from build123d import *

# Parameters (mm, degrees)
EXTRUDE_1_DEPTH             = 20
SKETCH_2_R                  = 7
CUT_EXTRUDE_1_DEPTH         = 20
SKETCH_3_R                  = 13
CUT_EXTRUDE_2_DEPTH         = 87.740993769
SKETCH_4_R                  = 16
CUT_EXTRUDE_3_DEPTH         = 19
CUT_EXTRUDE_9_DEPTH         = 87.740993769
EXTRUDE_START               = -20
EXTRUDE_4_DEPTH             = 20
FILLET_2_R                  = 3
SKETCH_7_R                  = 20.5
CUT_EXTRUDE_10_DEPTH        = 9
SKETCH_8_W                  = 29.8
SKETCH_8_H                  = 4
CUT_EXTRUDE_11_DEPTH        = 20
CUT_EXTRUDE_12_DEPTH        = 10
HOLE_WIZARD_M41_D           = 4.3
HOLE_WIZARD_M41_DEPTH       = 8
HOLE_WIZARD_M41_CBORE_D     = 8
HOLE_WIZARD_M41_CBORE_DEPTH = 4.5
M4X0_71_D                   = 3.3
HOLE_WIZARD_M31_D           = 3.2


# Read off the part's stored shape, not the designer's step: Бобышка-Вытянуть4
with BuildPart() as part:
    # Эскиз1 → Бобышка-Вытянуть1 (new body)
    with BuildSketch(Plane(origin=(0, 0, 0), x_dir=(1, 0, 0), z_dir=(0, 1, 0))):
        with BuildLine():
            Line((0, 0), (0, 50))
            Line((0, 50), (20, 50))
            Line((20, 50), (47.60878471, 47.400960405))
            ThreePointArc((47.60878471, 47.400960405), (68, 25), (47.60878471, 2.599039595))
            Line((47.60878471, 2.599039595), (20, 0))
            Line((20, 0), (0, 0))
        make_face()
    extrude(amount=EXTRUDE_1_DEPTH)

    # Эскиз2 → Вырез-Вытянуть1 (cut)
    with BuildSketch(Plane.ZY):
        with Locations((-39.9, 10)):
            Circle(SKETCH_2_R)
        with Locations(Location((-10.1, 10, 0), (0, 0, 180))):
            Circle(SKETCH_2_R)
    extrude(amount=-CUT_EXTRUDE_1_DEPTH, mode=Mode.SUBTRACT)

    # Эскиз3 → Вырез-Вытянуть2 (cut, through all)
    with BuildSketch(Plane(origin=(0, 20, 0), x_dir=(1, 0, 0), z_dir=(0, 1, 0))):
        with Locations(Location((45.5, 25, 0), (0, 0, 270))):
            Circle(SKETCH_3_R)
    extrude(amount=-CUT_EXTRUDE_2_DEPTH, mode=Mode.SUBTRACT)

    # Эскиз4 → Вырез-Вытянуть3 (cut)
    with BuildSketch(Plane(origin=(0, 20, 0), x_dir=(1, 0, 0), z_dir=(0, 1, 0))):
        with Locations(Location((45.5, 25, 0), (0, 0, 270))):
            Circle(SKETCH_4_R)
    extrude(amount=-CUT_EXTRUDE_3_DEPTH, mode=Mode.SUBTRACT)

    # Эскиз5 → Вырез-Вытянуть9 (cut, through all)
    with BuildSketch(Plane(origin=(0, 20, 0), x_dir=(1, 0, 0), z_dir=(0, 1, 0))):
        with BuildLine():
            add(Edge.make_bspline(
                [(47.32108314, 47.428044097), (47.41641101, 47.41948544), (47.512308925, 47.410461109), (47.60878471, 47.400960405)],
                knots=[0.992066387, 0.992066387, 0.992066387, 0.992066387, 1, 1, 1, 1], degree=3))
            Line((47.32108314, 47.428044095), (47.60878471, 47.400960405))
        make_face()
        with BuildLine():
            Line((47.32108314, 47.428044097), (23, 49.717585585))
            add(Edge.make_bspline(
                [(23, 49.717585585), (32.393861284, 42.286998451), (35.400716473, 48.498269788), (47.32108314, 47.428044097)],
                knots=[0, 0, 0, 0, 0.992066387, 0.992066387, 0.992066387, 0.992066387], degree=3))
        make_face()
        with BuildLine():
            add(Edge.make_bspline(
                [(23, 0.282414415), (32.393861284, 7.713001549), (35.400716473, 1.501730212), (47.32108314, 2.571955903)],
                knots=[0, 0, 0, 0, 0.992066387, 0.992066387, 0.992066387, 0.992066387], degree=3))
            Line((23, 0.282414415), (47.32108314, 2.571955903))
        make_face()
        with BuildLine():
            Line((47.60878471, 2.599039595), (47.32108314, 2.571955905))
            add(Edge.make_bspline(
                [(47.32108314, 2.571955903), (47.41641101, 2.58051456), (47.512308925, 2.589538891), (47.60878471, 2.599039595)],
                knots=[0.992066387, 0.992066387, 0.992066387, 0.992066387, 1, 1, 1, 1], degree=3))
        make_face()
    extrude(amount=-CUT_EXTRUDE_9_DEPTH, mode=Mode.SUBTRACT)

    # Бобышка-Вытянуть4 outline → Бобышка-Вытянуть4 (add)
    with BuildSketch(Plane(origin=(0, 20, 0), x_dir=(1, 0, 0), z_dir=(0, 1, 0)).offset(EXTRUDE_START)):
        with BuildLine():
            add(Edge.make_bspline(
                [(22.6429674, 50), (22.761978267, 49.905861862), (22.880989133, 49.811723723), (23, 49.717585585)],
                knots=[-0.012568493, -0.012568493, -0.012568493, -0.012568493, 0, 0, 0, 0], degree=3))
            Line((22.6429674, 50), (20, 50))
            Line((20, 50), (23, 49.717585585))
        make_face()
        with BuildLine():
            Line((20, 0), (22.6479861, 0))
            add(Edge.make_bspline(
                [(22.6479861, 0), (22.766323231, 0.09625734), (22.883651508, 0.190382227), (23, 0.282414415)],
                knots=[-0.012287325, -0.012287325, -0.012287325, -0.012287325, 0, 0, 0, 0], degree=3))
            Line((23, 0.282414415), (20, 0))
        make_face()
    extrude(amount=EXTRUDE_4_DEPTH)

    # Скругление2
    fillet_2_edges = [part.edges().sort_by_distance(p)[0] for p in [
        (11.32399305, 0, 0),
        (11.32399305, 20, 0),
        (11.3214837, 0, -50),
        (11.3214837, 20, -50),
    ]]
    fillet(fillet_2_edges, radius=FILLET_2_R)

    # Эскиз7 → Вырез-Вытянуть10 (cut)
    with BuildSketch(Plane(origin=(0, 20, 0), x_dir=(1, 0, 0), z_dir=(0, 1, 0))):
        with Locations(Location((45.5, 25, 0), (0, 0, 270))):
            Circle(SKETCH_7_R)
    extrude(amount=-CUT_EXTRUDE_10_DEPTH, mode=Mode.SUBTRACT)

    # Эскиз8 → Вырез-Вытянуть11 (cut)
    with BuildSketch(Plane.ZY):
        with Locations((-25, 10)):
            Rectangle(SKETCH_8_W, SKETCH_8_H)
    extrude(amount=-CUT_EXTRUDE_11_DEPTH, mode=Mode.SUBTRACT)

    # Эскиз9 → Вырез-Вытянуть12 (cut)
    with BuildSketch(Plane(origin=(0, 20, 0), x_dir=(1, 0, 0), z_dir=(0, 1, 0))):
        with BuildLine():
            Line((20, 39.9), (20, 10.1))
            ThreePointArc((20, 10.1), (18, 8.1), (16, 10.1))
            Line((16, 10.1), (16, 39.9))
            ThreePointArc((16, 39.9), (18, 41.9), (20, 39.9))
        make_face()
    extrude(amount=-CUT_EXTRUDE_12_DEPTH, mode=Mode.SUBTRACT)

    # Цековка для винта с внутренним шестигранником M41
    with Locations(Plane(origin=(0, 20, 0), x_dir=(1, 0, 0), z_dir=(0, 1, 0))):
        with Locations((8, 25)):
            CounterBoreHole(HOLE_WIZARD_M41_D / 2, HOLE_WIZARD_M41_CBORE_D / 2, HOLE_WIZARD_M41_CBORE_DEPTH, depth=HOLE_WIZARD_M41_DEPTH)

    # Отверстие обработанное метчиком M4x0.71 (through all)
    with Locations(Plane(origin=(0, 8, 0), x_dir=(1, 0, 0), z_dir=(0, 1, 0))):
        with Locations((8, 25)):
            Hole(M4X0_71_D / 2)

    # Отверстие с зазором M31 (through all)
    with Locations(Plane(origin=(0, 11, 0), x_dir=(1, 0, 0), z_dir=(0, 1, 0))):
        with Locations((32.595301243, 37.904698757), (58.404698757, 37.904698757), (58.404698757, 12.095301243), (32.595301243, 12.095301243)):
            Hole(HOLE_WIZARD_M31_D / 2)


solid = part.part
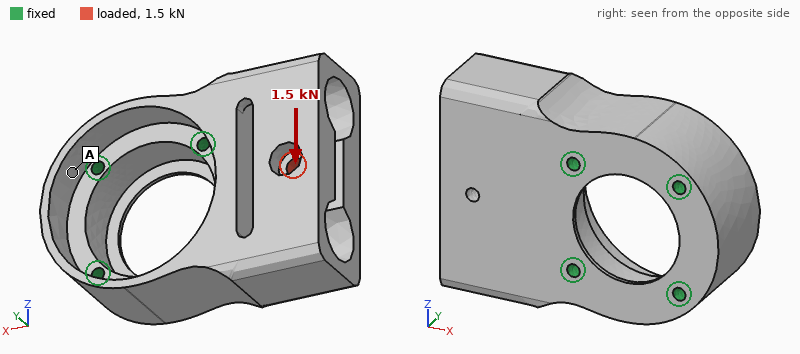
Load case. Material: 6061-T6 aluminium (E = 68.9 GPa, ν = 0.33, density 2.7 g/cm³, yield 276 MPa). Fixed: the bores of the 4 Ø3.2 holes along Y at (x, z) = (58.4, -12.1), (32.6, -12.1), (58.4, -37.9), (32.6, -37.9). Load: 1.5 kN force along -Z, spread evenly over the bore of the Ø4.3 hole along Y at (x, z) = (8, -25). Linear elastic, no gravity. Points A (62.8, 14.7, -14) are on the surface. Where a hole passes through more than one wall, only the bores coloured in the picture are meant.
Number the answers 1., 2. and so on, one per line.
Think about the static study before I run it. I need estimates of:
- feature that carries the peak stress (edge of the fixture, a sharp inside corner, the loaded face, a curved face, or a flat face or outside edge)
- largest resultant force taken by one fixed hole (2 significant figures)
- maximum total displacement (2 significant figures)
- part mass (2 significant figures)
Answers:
1. a curved face
2. 1.2 kN
3. 40 µm
4. 79 g
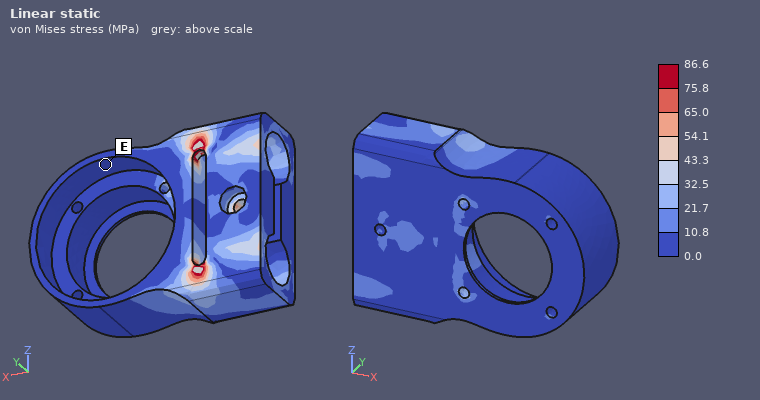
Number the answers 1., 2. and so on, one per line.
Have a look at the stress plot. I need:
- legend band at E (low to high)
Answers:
1. 0.0 to 10.8 MPa
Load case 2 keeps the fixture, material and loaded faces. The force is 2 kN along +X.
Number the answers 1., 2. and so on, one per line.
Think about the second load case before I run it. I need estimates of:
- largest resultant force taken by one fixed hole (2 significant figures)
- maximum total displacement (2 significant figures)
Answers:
1. 830 N
2. 91 µm
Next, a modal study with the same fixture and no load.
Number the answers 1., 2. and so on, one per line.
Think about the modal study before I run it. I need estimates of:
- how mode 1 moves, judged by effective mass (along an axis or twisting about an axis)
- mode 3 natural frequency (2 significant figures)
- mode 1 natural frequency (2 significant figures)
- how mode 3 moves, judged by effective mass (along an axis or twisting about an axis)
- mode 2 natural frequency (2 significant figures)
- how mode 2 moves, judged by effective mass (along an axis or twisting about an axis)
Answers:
1. along Y
2. 9800 Hz
3. 6000 Hz
4. along Z
5. 9300 Hz
6. twisting about X
